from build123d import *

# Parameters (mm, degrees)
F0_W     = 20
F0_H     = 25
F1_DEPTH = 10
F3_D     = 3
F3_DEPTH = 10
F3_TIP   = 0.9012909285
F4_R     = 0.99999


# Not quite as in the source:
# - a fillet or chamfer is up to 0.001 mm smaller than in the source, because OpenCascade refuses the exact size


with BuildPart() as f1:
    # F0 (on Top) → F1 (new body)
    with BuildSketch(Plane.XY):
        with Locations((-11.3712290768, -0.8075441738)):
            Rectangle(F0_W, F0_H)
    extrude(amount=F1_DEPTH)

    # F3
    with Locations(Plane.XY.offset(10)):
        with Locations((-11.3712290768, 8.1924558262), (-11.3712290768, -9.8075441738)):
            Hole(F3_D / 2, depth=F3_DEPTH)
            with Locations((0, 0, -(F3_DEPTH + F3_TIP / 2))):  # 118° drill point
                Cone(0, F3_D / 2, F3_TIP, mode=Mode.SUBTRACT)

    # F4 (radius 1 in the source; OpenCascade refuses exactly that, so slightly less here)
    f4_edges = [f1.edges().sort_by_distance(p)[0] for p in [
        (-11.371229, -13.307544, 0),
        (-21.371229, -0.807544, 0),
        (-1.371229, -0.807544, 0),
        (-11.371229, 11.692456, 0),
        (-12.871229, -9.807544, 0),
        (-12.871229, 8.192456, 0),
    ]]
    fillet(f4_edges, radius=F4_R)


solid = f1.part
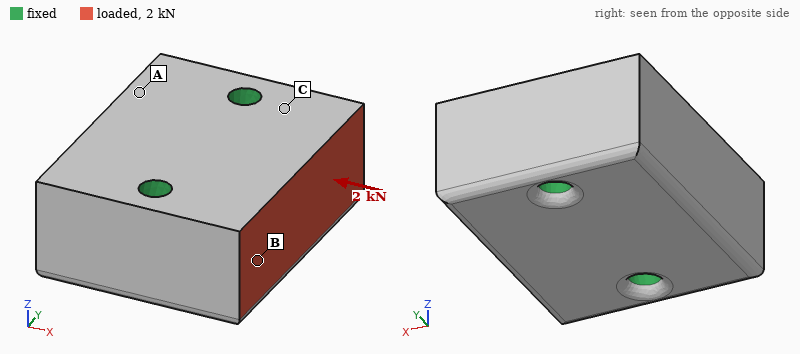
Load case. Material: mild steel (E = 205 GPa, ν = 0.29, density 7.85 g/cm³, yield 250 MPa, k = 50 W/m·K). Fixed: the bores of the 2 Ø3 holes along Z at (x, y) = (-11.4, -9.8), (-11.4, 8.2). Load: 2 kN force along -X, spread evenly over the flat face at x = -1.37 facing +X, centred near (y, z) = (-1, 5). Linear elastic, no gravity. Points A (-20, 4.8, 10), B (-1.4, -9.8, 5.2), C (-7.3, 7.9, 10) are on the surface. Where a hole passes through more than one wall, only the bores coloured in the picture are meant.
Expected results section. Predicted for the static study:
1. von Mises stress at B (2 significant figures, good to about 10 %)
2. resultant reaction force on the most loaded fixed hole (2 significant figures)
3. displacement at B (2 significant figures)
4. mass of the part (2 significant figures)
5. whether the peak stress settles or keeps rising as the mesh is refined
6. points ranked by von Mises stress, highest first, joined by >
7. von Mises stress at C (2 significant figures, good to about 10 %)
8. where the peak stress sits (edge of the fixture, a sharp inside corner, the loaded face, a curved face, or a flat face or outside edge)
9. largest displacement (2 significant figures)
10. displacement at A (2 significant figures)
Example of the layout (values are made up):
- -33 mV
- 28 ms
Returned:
- 8.4 MPa
- 1.0 kN
- 0.47 µm
- 38 g
- keeps rising
- C > B > A
- 14 MPa
- edge of the fixture
- 0.70 µm
- 0.18 µm
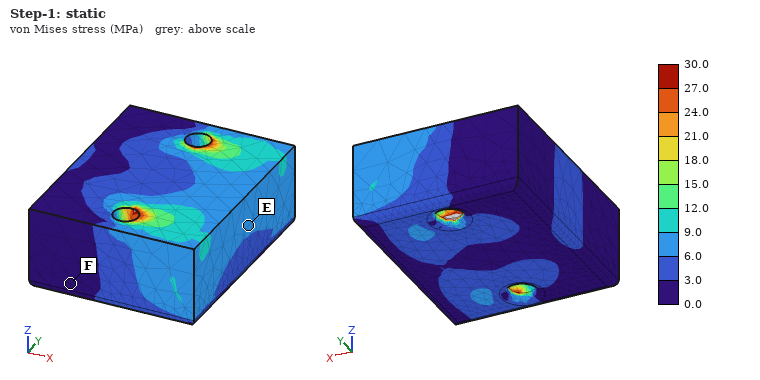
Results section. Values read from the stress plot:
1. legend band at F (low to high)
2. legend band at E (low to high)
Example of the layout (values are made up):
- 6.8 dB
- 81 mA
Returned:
- 0.0 to 3.0 MPa
- 6.0 to 9.0 MPa
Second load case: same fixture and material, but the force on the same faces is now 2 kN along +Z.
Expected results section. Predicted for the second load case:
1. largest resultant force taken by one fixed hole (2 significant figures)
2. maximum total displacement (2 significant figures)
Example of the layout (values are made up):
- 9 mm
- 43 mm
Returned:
- 1.0 kN
- 4.6 µm
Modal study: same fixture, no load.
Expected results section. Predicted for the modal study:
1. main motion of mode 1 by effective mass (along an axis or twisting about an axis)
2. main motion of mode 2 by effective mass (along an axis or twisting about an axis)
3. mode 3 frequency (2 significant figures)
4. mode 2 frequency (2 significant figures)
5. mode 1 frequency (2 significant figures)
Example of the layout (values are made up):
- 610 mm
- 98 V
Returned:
- twisting about Y
- along Z
- 64 kHz
- 47 kHz
- 40 kHz
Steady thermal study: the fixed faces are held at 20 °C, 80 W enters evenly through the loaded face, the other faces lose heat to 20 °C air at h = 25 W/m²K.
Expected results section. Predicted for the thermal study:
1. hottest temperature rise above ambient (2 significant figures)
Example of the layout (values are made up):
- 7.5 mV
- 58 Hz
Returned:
- 75 K
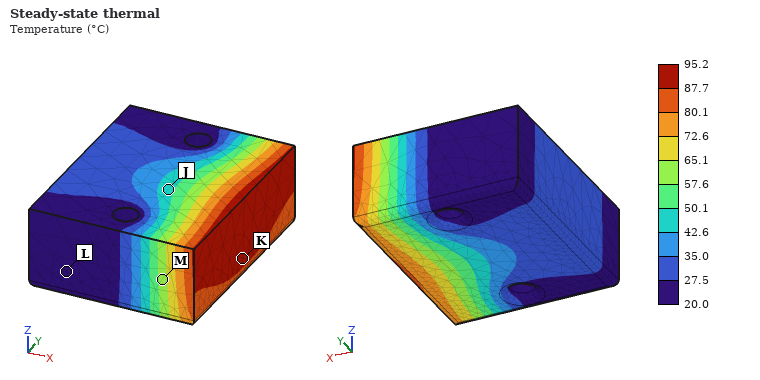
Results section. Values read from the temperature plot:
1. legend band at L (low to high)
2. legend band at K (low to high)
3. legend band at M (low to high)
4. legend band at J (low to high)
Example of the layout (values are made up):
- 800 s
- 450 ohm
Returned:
- 20.0 to 27.5 °C
- 87.7 to 95.2 °C
- 57.6 to 65.1 °C
- 42.6 to 50.1 °C
